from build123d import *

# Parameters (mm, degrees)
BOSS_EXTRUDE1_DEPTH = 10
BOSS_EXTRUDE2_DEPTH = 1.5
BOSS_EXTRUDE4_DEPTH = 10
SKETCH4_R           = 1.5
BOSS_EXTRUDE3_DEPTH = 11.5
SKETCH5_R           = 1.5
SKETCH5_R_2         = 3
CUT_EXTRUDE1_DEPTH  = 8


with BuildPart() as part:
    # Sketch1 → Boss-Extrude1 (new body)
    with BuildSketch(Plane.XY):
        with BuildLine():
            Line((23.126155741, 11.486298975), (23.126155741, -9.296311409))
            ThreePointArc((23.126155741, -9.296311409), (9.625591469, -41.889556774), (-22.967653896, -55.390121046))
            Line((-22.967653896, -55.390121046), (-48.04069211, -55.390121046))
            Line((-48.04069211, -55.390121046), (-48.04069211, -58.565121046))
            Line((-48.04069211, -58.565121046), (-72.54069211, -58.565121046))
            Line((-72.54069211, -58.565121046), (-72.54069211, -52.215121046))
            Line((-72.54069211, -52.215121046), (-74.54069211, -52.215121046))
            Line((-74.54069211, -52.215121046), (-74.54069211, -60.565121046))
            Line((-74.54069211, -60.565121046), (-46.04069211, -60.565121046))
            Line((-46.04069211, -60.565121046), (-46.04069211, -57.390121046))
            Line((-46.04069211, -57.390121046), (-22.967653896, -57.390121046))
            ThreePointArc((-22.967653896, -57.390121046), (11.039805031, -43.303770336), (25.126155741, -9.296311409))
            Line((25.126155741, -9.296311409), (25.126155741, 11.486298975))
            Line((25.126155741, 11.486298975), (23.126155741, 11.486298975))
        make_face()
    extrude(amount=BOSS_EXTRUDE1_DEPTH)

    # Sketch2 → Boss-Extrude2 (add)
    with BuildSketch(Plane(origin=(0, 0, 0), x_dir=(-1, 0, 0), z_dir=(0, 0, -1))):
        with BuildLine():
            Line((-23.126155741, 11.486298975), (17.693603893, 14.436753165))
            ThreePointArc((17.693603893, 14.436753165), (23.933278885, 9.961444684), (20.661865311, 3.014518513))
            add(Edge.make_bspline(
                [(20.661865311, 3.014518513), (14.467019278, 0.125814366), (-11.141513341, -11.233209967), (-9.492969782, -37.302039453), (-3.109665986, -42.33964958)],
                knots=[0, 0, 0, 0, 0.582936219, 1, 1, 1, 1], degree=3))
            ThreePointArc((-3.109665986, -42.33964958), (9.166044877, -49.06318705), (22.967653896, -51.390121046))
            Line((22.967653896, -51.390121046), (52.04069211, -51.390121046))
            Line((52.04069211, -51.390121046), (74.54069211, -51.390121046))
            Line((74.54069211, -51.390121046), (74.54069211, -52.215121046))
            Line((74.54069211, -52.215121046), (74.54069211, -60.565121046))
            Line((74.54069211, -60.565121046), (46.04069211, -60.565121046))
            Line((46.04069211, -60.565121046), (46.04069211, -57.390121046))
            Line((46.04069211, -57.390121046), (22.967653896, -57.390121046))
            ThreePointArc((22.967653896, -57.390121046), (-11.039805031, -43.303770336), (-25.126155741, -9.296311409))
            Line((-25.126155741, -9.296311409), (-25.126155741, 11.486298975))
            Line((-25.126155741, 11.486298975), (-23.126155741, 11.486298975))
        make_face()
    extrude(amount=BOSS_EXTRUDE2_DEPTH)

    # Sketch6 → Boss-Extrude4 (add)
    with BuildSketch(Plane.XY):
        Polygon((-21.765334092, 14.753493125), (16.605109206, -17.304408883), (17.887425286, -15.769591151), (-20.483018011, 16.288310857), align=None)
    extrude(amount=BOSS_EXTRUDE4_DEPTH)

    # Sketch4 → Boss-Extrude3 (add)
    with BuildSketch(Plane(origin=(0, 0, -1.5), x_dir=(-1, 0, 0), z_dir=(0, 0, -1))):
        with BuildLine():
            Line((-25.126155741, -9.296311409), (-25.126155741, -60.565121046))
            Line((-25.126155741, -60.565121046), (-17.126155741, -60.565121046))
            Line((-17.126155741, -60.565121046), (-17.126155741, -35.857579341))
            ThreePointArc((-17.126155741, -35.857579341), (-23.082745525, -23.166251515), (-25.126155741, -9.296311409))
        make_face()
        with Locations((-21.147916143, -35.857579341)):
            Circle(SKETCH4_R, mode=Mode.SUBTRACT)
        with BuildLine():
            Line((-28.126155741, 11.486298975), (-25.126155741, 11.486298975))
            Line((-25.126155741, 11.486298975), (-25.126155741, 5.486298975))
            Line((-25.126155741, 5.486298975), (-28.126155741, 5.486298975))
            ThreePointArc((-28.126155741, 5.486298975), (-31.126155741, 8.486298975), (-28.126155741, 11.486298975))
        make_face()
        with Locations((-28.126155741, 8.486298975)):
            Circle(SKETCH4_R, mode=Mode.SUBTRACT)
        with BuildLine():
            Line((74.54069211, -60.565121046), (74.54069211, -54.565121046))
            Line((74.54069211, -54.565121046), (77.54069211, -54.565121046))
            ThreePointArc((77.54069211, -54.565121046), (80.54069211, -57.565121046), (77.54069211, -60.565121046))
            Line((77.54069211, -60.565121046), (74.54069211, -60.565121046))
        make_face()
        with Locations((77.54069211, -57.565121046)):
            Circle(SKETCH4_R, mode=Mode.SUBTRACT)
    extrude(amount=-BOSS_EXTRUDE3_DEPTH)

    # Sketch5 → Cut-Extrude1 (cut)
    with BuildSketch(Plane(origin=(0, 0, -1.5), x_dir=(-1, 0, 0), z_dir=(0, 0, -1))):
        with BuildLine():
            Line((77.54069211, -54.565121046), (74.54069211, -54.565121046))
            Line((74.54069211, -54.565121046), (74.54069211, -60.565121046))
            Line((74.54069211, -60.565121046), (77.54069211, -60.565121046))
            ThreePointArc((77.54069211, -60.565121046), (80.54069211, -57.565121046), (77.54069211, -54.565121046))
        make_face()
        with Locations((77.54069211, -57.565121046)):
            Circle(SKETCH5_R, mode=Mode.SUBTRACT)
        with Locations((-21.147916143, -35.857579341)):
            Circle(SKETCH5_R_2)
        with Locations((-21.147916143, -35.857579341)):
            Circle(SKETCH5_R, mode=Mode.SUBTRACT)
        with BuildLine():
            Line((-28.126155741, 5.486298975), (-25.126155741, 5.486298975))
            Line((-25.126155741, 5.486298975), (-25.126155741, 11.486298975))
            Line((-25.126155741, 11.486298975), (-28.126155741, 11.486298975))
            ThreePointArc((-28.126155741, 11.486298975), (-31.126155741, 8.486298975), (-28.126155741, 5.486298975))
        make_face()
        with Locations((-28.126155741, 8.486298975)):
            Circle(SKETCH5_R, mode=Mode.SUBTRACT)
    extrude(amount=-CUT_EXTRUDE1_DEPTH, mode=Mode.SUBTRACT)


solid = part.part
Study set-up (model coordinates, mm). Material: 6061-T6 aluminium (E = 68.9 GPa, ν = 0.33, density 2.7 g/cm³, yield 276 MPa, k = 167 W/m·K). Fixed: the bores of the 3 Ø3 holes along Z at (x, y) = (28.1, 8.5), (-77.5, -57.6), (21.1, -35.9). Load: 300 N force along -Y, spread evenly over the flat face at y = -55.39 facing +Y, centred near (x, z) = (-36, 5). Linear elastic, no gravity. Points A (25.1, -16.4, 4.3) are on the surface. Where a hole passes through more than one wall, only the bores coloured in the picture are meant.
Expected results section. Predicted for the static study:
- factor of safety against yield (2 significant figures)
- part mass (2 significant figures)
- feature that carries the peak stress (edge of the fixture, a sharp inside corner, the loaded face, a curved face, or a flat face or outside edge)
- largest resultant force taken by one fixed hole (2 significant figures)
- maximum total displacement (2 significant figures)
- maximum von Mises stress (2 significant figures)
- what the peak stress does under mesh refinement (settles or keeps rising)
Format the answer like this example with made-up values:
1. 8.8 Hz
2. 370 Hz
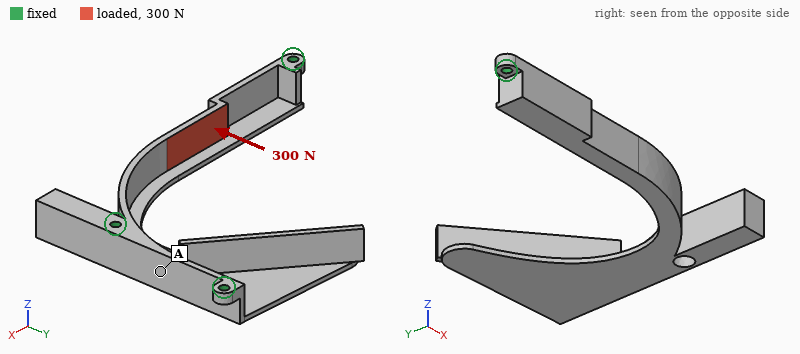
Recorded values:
1. 1.4
2. 27 g
3. a flat face or outside edge
4. 350 N
5. 0.46 mm
6. 190 MPa
7. settles
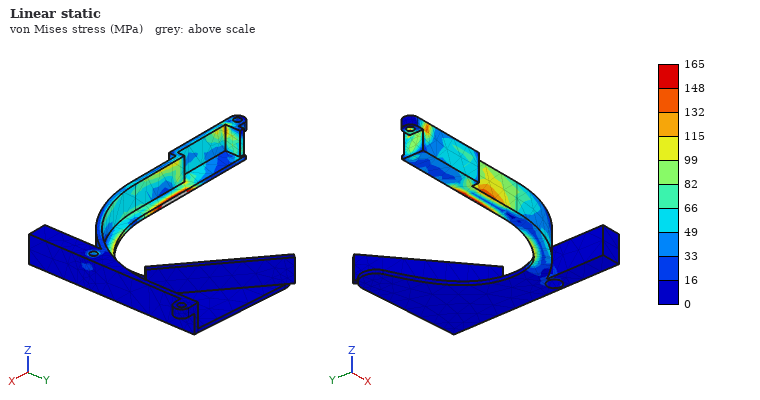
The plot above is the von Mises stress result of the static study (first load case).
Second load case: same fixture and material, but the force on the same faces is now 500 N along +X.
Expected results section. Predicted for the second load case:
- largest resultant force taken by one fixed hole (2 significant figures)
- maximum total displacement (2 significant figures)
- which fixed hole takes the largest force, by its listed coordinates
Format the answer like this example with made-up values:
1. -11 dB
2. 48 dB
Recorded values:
1. 480 N
2. 0.12 mm
3. (-77.5, -57.6)
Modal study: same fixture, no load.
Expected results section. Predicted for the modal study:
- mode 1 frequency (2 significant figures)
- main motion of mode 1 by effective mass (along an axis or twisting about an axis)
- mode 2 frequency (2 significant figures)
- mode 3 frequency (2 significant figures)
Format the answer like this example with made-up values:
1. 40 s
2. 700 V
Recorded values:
1. 720 Hz
2. along Z
3. 2500 Hz
4. 2800 Hz
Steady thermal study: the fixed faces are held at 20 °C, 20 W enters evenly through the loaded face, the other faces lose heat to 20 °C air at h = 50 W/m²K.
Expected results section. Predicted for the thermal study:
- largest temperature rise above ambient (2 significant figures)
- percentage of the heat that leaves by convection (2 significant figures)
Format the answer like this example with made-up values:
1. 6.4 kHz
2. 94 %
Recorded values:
1. 73 K
2. 35 %
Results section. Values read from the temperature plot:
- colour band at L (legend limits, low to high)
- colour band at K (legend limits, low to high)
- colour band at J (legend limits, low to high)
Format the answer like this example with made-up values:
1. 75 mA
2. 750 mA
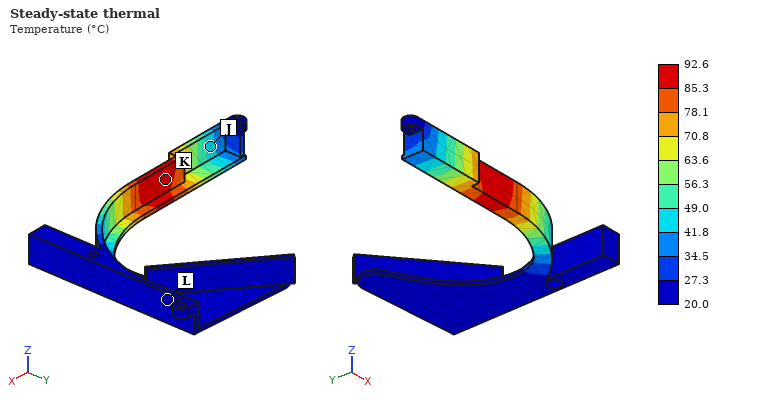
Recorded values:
1. 20.0 to 27.3 °C
2. 85.3 to 92.6 °C
3. 41.8 to 49.0 °C
